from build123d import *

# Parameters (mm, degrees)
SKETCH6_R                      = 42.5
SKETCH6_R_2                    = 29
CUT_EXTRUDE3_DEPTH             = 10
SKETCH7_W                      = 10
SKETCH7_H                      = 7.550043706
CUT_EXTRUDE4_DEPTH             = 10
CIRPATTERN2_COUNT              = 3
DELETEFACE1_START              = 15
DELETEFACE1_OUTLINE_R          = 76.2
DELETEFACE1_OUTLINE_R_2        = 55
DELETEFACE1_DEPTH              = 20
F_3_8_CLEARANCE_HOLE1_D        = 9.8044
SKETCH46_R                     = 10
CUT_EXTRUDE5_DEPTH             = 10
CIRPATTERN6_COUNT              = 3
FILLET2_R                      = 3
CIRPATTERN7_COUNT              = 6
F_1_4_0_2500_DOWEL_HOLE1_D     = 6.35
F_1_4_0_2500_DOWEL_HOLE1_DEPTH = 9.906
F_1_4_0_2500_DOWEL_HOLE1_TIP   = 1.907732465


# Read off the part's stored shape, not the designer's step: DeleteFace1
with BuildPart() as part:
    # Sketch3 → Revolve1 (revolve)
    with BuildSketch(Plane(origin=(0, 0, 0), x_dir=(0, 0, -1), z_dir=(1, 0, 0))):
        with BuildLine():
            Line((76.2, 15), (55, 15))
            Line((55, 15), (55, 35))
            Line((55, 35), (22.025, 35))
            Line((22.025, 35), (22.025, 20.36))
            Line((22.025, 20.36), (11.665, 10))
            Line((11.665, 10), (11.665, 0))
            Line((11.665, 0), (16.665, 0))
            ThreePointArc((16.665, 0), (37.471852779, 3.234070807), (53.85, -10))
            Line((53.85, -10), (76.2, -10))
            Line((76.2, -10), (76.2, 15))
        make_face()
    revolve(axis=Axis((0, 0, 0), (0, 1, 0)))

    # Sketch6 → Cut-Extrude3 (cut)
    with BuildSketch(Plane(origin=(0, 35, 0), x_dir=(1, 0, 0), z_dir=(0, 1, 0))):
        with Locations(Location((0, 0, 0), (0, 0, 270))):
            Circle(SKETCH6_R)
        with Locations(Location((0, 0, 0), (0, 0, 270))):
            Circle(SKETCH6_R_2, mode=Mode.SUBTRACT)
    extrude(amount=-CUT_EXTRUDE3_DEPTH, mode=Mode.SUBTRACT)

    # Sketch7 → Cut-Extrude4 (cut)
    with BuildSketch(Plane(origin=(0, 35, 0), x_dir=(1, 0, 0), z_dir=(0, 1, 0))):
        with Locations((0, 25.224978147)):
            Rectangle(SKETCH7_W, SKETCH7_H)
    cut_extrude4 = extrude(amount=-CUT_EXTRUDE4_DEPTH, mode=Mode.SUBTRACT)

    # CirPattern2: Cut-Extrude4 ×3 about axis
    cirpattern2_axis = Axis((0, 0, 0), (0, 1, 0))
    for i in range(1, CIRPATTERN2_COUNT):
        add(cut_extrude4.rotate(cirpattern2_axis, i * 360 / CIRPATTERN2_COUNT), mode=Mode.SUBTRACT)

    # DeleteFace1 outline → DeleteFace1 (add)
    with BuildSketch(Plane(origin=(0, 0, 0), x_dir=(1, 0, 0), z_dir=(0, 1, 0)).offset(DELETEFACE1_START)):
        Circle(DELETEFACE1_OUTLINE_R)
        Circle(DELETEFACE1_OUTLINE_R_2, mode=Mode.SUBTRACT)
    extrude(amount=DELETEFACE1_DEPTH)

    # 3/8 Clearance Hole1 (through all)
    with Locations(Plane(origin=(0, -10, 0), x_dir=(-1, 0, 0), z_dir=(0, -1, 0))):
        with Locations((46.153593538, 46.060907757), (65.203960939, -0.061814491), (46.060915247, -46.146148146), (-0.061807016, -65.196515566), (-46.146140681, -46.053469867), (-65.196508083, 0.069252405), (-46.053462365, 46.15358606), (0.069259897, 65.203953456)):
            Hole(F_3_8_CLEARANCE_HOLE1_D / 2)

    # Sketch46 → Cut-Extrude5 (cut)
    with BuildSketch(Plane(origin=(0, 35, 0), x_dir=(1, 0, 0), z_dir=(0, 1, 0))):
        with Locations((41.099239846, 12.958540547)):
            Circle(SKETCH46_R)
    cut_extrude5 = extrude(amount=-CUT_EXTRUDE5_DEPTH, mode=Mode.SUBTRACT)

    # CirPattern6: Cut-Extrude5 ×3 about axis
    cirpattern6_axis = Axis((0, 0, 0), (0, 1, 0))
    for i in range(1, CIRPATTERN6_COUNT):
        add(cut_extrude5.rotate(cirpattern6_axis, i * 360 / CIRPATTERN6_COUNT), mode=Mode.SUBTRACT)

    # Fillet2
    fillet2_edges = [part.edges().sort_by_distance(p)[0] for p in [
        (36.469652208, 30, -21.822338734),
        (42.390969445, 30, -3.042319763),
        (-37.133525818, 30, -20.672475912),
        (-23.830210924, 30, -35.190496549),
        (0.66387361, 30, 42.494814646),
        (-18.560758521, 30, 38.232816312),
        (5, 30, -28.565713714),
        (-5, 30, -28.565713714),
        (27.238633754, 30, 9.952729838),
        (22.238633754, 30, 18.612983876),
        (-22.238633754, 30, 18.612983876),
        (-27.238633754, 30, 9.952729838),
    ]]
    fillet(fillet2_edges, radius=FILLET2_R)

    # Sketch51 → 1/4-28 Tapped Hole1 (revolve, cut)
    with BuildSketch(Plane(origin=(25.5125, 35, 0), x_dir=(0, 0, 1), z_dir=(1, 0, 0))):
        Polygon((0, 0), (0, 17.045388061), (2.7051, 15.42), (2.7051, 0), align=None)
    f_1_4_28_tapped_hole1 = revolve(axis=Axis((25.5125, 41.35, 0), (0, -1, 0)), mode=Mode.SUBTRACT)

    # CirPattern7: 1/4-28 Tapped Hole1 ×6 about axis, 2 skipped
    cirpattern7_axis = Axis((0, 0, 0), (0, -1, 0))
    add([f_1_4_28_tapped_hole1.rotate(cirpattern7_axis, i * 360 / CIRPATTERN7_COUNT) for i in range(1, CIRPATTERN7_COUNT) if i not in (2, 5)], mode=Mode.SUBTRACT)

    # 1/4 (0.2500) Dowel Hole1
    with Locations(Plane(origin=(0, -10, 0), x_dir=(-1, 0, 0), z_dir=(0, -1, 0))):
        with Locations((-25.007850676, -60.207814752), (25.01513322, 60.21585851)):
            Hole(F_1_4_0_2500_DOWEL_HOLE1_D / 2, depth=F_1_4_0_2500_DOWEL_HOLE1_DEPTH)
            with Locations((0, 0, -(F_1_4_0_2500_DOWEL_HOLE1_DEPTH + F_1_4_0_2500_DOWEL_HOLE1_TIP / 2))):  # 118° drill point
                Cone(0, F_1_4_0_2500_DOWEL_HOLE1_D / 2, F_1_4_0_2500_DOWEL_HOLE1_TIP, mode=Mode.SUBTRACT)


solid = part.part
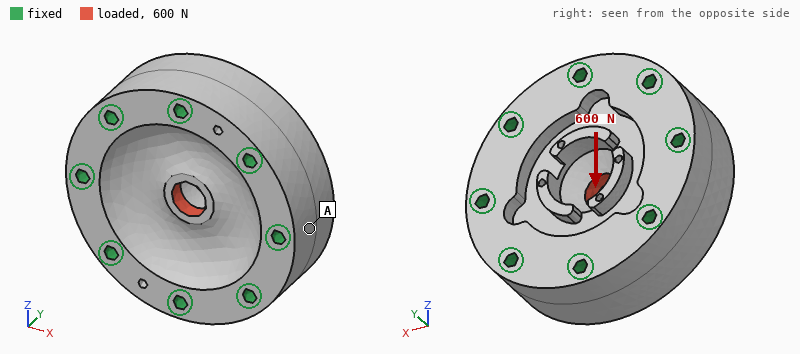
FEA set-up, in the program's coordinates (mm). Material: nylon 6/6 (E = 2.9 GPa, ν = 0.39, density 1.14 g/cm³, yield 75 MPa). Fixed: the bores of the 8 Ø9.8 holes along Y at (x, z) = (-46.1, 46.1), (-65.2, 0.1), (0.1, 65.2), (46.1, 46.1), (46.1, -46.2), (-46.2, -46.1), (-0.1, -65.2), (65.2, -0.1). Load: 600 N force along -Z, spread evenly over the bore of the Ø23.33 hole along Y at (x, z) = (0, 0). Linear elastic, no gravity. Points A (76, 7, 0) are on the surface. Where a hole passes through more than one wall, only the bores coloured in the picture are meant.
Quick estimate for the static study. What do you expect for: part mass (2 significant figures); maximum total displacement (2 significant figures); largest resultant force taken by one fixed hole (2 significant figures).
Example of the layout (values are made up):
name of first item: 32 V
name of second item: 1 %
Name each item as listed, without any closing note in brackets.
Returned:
part mass: 710 g
maximum total displacement: 11 µm
largest resultant force taken by one fixed hole: 140 N
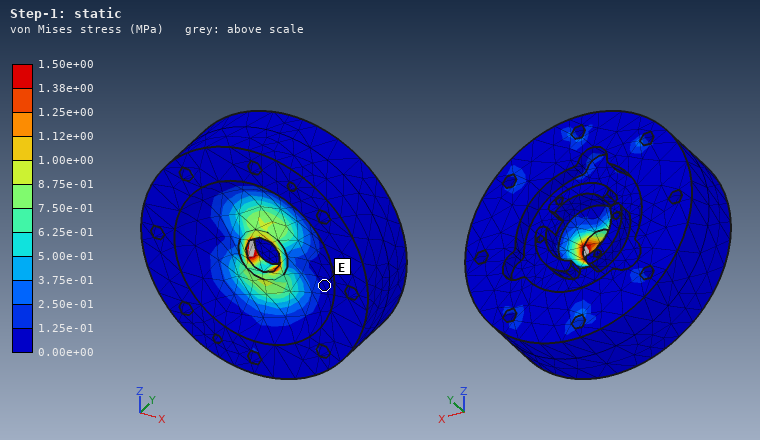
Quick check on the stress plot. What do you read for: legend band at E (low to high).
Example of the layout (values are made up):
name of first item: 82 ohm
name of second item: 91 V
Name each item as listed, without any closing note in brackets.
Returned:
legend band at E: 0.00e+00 to 1.25e-01 MPa
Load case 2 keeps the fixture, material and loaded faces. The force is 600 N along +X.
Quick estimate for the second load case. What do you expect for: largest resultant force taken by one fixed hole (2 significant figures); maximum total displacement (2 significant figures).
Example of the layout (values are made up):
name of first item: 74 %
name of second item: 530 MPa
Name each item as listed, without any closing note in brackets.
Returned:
largest resultant force taken by one fixed hole: 140 N
maximum total displacement: 10 µm
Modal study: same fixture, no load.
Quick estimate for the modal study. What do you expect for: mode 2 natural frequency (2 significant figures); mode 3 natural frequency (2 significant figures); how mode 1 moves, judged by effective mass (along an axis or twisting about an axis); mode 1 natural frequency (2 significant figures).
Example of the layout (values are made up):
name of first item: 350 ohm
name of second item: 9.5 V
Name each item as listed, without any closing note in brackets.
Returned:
mode 2 natural frequency: 6000 Hz
mode 3 natural frequency: 6000 Hz
how mode 1 moves, judged by effective mass: along Y
mode 1 natural frequency: 4500 Hz
